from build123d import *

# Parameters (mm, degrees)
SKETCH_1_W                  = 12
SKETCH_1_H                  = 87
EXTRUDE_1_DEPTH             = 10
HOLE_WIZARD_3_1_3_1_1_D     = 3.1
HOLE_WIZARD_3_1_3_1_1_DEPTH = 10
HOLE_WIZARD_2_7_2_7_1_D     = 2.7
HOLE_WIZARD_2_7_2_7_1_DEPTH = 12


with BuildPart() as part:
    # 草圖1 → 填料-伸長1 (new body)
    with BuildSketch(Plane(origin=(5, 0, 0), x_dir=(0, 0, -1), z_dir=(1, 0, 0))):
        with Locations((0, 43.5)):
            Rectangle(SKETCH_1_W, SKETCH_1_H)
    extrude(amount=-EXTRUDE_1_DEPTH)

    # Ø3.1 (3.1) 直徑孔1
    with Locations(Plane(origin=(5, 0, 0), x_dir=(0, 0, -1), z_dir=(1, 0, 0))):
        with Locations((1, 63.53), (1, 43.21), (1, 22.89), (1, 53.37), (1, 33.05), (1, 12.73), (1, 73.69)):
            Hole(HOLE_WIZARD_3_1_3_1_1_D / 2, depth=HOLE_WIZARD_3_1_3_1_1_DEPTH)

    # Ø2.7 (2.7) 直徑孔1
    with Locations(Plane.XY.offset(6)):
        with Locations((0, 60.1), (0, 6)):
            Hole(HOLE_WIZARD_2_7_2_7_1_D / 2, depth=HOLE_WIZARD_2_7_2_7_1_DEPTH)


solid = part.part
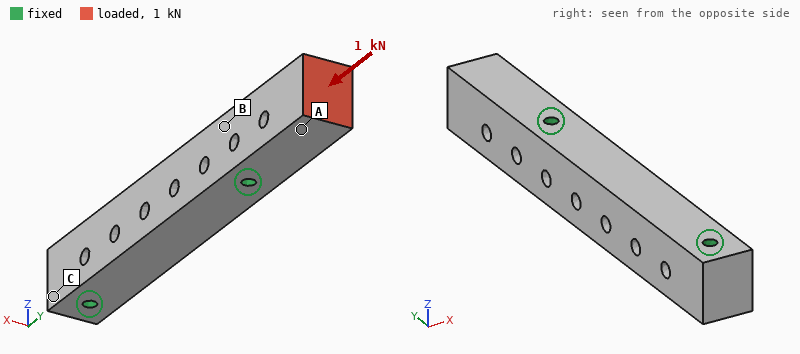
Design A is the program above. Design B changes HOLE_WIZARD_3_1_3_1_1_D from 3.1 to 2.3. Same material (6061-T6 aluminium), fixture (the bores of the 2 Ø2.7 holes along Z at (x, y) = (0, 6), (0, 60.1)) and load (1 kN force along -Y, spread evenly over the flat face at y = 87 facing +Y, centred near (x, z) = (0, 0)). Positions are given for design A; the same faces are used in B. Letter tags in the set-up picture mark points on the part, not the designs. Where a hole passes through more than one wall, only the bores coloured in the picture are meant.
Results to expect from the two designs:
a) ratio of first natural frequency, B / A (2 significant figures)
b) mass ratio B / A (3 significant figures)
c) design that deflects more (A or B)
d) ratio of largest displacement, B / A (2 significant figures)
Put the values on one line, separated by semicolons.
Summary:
1.0; 1.02; A; 0.92
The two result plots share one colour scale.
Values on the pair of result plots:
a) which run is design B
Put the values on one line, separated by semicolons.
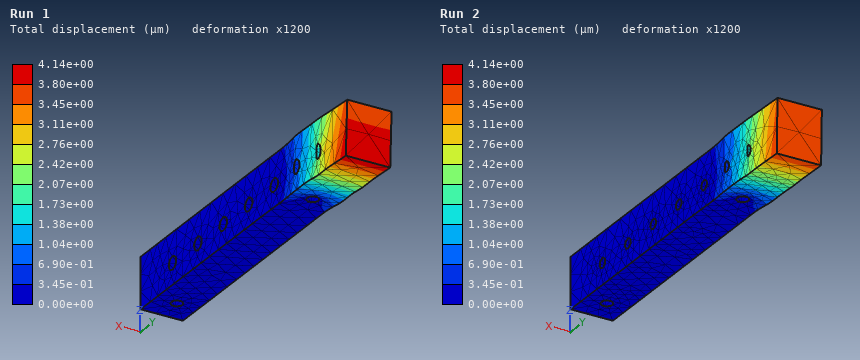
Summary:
Run 2
